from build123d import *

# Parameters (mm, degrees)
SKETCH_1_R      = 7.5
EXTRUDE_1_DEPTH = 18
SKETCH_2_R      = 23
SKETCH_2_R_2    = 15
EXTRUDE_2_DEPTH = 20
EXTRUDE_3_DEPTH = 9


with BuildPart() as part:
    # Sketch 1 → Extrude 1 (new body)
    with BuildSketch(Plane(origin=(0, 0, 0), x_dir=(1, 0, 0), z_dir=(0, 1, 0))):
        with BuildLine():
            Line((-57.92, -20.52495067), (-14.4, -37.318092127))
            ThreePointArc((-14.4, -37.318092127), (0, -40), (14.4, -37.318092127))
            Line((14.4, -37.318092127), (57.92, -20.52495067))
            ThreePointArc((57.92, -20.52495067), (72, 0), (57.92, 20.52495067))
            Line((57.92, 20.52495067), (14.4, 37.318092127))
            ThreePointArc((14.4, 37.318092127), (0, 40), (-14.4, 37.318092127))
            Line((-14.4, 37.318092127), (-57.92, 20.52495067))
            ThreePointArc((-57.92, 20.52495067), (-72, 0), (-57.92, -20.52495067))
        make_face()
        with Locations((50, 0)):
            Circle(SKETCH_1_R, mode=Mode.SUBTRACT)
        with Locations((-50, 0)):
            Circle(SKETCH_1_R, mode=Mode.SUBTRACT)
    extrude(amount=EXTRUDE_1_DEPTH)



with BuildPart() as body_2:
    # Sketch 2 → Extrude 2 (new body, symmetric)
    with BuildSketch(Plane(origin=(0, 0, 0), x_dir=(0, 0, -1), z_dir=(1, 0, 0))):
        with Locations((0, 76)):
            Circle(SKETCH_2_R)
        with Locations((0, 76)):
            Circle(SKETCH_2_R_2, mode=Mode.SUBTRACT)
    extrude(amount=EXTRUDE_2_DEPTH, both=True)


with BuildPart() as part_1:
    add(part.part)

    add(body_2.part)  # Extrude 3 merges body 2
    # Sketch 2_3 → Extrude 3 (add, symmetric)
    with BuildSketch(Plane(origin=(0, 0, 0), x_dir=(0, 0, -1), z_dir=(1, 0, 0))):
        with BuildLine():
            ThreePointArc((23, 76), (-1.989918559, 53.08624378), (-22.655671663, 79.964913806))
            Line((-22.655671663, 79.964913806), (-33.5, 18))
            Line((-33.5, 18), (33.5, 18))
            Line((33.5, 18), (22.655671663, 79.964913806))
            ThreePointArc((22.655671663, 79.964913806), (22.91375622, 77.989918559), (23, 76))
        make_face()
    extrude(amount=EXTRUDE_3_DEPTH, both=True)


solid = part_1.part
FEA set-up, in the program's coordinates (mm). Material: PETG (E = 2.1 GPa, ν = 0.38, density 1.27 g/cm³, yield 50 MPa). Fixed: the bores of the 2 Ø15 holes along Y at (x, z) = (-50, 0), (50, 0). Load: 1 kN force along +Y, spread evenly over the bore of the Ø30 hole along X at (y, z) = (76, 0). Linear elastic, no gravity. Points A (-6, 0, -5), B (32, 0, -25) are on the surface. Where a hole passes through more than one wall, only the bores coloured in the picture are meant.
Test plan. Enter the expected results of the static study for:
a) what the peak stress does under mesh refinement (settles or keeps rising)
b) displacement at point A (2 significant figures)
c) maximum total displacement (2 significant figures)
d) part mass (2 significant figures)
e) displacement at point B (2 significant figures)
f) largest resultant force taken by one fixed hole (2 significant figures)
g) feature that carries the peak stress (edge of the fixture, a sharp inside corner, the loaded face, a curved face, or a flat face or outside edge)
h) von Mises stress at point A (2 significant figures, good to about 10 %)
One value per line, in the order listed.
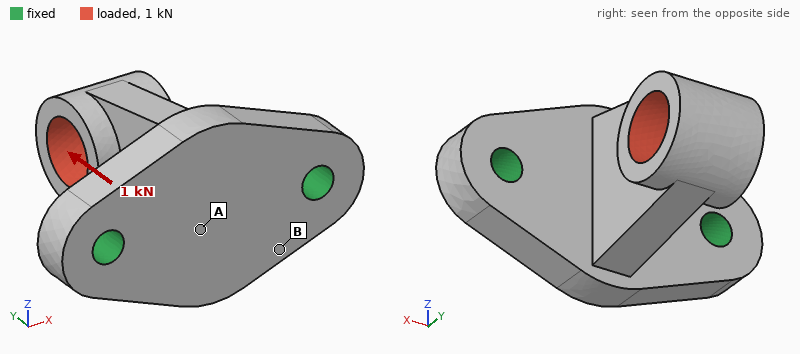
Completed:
keeps rising
0.085 mm
0.15 mm
280 g
0.047 mm
500 N
edge of the fixture
2.2 MPa
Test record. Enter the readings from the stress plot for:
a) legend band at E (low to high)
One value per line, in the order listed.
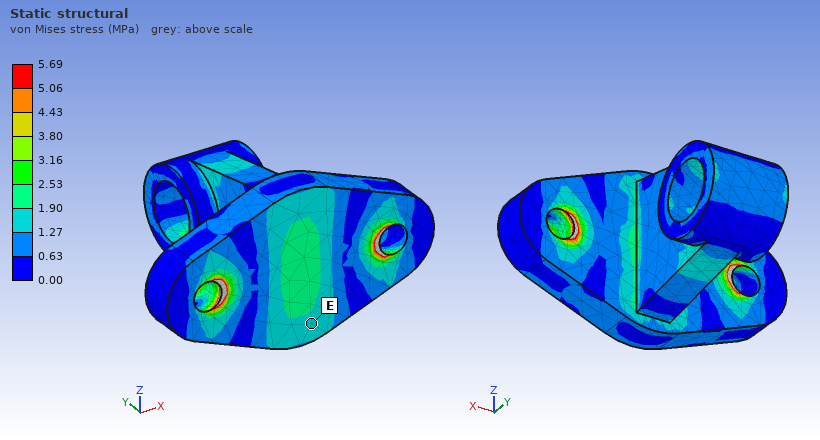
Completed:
1.27 to 1.90 MPa
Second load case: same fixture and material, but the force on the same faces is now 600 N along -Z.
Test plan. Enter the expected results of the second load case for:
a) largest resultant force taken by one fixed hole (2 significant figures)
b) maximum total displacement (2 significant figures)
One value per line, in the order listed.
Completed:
300 N
0.98 mm
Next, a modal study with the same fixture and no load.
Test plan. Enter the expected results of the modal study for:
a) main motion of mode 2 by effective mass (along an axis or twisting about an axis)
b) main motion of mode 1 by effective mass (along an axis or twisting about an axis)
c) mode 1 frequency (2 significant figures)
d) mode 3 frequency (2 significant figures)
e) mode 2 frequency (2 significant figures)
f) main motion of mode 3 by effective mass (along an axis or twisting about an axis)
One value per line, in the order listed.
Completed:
along Z
along X
500 Hz
1200 Hz
540 Hz
along Y
